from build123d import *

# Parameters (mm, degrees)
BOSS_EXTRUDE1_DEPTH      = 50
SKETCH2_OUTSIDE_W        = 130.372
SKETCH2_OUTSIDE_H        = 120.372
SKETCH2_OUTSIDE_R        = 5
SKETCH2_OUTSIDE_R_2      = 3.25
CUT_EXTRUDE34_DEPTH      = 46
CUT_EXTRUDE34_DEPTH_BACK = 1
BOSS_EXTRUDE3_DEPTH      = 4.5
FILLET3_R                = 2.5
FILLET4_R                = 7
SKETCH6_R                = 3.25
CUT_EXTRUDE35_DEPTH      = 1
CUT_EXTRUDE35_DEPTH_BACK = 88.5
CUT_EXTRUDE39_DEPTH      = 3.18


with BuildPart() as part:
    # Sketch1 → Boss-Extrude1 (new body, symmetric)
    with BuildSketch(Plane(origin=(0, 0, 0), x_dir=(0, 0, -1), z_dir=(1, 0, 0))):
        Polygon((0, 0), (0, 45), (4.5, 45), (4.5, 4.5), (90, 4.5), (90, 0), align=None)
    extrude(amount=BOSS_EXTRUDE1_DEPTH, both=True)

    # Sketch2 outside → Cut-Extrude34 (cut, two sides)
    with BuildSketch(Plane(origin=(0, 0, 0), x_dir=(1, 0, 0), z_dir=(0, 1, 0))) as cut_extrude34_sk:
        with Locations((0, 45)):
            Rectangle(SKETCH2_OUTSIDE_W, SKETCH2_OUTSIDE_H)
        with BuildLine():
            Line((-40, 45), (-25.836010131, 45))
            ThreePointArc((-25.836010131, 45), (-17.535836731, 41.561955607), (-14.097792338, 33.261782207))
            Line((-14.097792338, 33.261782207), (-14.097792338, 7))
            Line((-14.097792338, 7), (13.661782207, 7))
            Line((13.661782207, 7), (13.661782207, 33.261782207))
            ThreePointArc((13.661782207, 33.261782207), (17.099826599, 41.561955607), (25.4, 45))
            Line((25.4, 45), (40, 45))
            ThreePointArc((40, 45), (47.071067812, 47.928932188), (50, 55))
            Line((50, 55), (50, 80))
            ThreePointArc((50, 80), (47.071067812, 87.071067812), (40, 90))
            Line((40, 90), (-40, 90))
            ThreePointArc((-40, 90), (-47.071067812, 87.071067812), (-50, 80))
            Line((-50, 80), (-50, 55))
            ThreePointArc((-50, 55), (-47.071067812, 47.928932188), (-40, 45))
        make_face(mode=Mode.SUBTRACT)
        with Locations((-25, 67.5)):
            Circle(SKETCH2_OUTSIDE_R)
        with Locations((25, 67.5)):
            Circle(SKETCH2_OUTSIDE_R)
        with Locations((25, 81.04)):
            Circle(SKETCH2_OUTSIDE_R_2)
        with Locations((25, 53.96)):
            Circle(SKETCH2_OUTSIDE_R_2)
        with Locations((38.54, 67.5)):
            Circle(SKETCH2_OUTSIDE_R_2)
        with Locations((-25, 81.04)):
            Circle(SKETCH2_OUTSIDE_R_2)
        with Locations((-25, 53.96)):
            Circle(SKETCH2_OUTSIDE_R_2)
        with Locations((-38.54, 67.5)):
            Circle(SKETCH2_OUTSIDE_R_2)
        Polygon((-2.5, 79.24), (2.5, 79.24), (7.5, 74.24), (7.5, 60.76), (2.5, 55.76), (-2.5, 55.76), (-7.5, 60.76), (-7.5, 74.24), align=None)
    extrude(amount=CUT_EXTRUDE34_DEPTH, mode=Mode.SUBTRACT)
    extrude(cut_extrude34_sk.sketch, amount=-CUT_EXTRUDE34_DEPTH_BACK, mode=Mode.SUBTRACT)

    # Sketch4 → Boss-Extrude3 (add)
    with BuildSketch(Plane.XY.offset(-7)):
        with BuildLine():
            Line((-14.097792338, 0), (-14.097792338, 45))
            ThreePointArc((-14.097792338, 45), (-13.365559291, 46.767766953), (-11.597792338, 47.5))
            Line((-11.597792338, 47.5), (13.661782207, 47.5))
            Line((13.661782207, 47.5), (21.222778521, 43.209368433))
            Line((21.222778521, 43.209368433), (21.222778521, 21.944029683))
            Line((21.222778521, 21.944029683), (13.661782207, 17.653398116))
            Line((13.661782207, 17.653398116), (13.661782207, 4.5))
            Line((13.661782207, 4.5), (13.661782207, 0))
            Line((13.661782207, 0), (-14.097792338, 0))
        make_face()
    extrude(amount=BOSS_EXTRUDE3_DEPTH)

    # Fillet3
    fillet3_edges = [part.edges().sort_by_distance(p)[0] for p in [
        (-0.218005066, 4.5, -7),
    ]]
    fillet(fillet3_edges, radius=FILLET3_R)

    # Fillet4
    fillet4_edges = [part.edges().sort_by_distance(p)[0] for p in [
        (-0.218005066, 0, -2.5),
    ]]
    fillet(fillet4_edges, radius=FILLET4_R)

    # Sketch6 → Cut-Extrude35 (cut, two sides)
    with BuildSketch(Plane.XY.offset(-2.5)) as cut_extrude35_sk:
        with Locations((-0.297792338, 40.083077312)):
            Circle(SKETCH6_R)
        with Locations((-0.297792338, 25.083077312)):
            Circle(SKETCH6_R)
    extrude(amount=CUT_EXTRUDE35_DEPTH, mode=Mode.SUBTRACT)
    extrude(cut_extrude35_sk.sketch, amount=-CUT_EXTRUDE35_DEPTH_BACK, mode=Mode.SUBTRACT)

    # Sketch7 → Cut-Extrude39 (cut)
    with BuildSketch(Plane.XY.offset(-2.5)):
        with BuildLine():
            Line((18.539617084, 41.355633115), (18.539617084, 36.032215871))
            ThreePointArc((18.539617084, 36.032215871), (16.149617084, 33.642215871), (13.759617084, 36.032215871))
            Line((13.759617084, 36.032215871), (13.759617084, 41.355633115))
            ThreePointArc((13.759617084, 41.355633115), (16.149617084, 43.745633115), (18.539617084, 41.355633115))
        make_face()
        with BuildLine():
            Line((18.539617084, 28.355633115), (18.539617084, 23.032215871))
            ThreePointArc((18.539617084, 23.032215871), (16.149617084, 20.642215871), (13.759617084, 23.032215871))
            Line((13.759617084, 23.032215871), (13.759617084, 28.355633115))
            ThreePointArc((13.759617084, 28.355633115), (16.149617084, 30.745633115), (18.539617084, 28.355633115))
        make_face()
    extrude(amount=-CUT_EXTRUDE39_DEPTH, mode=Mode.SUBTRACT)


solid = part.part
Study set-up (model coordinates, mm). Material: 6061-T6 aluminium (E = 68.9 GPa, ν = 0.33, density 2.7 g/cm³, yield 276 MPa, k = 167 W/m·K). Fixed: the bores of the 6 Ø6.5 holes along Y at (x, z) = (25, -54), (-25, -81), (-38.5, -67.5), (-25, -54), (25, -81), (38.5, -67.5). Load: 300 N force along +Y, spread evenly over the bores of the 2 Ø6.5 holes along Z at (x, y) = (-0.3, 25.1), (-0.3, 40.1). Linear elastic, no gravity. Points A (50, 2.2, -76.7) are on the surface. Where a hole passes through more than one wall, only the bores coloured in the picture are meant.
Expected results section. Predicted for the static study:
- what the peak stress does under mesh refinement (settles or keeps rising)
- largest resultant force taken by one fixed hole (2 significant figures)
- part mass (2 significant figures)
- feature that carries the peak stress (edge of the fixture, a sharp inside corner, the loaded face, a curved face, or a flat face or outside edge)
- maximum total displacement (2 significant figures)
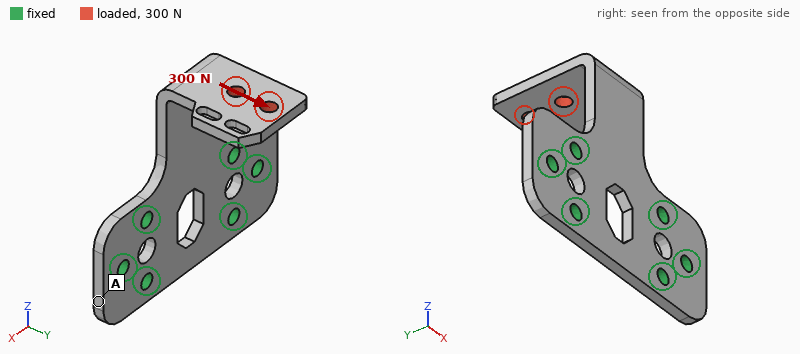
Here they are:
keeps rising
270 N
75 g
edge of the fixture
1.4 mm
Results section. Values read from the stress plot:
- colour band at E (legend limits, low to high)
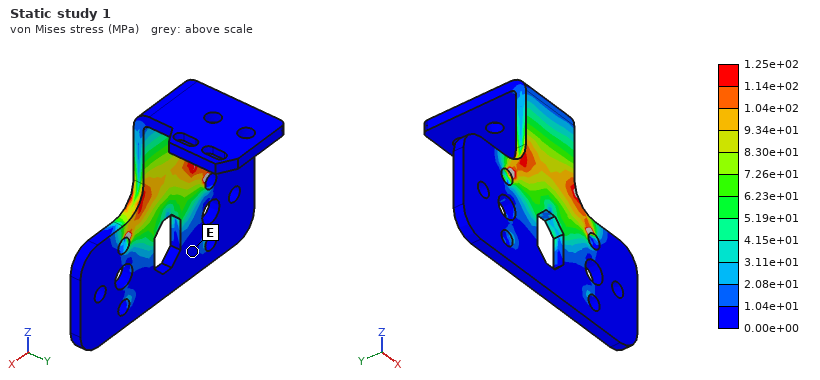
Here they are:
0.00e+00 to 1.04e+01 MPa
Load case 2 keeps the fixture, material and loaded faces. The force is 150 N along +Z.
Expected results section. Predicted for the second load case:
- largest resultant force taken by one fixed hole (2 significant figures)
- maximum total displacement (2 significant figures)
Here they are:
69 N
0.89 mm
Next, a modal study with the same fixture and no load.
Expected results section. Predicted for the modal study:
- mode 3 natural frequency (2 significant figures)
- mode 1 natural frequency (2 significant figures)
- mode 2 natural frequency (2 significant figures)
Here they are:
1500 Hz
550 Hz
1000 Hz
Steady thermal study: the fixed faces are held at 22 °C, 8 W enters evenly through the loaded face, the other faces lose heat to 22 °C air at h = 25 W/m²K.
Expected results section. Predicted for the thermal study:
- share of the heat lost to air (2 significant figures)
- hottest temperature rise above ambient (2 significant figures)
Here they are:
29 %
24 K
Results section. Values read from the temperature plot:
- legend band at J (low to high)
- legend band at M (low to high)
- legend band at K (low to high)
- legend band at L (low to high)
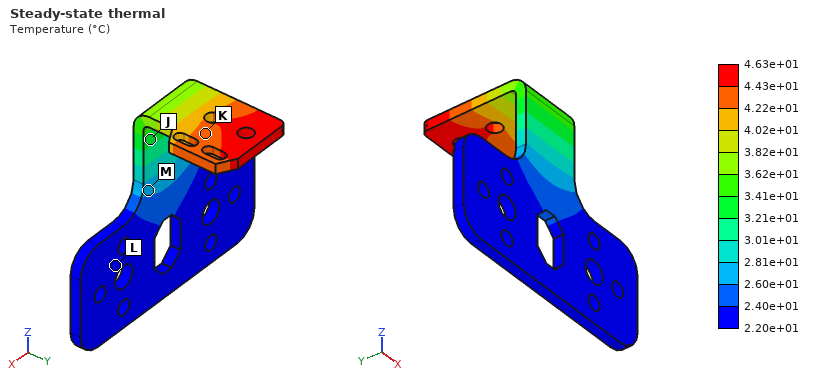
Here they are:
3.21e+01 to 3.41e+01 °C
2.60e+01 to 2.81e+01 °C
4.22e+01 to 4.43e+01 °C
2.20e+01 to 2.40e+01 °C
